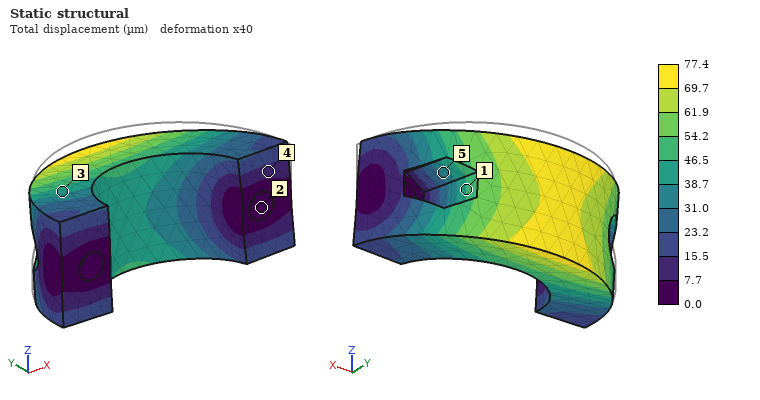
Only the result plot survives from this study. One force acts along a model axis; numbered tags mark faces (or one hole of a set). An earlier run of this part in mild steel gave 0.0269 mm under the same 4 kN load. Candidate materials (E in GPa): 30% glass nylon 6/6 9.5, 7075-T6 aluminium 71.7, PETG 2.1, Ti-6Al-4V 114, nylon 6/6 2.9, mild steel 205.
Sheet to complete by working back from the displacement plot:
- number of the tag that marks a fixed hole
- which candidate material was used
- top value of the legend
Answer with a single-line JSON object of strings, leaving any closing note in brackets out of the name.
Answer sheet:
{"number of the tag that marks a fixed hole": "2", "which candidate material was used": "7075-T6 aluminium", "top value of the legend": "77.4 µm"}
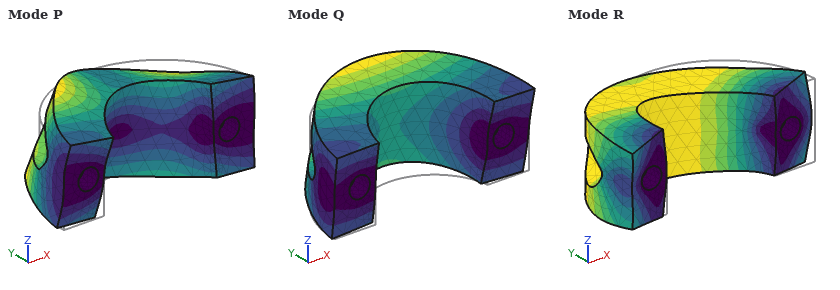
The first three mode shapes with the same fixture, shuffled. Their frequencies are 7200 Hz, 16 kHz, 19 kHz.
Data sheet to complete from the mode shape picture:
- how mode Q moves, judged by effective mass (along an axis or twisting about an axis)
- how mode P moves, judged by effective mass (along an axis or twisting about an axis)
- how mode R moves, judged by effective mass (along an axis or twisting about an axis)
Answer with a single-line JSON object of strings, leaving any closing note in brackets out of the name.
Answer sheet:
{"how mode Q moves, judged by effective mass": "along Z", "how mode P moves, judged by effective mass": "twisting about Y", "how mode R moves, judged by effective mass": "along X"}
